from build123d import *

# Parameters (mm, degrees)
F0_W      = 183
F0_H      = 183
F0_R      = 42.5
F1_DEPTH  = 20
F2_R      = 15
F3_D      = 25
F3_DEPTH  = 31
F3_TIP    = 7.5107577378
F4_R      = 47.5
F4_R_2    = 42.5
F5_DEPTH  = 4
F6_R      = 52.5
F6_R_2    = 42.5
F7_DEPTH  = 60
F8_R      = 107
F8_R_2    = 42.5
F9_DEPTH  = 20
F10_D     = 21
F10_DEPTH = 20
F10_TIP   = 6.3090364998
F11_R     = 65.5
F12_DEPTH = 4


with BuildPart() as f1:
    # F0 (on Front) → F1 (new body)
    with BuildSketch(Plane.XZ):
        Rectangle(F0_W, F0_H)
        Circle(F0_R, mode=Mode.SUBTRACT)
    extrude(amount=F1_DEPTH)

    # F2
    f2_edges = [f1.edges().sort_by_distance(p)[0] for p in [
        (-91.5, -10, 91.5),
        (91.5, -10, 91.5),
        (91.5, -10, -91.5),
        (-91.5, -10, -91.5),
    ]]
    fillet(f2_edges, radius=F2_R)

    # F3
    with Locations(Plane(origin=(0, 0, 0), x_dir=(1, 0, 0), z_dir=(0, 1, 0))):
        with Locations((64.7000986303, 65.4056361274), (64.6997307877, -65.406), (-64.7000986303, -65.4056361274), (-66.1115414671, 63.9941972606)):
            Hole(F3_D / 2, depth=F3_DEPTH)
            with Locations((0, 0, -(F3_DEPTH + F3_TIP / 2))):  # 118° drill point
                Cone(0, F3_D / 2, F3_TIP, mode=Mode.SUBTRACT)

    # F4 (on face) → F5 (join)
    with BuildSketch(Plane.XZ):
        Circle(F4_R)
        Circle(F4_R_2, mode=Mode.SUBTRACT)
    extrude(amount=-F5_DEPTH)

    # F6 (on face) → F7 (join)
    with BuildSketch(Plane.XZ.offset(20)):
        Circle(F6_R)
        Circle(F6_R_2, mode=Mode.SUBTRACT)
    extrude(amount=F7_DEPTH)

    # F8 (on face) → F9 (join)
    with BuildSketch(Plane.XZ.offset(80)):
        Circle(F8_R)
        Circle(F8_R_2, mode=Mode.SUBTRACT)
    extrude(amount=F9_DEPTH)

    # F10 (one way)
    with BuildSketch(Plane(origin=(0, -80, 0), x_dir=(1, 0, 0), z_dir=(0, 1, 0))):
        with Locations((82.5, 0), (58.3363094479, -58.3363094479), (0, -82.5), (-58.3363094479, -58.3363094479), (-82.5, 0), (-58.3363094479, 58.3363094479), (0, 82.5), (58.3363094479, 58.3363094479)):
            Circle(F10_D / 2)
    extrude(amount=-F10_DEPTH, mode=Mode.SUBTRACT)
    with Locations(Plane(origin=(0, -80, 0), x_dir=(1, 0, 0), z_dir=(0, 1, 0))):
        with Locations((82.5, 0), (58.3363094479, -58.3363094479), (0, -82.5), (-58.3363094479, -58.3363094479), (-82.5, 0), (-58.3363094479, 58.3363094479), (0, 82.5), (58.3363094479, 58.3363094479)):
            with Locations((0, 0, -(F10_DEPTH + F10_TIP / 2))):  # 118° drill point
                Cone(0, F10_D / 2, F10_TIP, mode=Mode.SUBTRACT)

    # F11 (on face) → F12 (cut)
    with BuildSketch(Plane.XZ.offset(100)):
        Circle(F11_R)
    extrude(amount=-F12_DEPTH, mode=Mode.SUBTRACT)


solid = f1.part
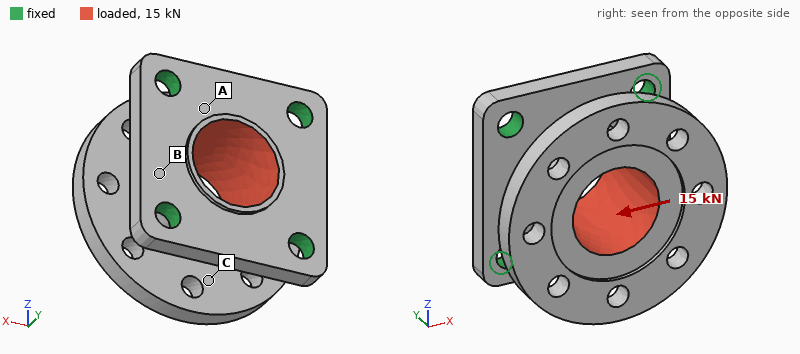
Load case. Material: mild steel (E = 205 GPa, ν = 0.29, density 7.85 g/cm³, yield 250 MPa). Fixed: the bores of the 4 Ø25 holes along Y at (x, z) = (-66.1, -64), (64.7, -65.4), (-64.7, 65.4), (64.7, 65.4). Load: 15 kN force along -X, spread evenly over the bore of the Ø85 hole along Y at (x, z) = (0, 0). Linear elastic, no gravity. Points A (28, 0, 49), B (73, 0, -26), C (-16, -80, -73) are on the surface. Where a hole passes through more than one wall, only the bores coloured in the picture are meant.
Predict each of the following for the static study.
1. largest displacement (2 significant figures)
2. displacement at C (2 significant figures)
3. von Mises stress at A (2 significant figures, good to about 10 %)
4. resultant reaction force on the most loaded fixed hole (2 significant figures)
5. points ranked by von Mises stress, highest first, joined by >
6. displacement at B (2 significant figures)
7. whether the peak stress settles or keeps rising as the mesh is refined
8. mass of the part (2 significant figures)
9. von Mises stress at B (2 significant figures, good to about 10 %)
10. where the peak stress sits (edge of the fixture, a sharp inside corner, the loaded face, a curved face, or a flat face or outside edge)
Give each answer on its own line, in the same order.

15 µm
9.6 µm
2.5 MPa
4.7 kN
B > A > C
2.3 µm
keeps rising
9.6 kg
4.2 MPa
edge of the fixture
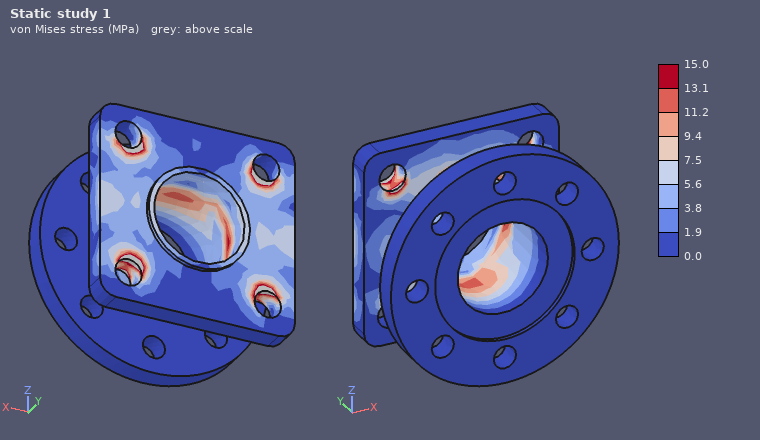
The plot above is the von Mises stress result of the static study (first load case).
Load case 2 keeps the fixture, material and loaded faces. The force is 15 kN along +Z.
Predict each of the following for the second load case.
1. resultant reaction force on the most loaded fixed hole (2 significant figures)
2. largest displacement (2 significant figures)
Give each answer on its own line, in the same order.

4.7 kN
14 µm
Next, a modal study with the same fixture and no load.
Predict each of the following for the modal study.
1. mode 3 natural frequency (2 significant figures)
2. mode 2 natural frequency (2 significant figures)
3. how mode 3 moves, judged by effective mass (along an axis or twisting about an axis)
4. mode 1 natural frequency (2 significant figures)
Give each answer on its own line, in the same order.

2000 Hz
1400 Hz
along Y
1400 Hz
